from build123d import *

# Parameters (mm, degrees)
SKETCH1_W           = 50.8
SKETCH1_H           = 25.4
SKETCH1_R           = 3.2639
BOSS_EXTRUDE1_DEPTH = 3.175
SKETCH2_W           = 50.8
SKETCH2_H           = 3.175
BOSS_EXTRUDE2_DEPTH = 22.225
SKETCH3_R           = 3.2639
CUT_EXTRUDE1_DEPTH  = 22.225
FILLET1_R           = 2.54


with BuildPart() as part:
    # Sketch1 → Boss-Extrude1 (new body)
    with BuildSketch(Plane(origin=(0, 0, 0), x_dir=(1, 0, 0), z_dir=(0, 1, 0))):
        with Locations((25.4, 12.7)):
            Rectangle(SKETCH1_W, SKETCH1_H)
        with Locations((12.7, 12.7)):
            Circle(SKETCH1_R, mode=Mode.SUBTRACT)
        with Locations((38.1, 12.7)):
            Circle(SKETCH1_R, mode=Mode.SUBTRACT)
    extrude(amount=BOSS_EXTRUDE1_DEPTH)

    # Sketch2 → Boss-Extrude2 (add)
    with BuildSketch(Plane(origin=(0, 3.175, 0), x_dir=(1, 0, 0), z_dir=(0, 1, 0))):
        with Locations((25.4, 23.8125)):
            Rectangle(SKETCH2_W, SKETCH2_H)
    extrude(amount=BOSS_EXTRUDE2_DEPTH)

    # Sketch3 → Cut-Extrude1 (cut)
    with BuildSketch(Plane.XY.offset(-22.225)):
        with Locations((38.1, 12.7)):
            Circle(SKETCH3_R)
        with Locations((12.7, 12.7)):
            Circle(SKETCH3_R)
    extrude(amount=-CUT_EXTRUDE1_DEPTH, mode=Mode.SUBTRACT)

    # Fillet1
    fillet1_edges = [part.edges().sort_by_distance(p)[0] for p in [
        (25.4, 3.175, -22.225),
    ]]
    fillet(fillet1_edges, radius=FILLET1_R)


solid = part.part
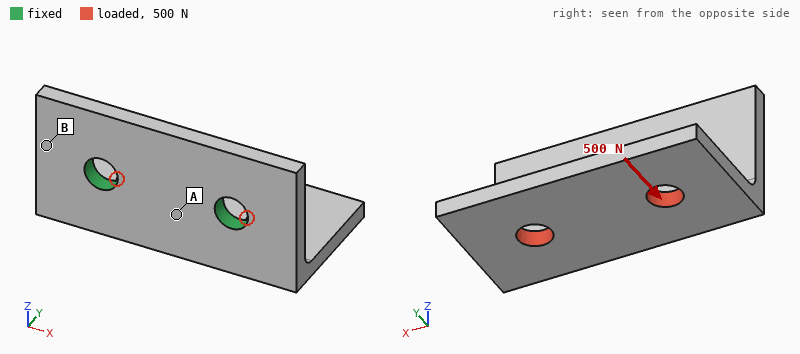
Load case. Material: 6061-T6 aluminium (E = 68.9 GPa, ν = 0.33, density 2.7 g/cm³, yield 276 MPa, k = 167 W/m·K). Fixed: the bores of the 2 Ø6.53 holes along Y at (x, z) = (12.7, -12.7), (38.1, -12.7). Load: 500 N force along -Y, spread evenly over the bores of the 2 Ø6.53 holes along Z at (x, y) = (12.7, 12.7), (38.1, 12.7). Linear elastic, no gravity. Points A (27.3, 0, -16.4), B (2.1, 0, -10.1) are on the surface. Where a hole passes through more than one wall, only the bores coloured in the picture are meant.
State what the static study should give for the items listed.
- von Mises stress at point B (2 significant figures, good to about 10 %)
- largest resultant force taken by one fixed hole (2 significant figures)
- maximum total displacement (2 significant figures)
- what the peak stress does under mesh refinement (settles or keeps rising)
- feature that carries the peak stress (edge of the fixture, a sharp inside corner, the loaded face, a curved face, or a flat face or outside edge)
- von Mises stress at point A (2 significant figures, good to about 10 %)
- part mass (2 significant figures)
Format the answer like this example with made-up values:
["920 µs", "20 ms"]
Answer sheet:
["9.0 MPa", "250 N", "61 µm", "keeps rising", "edge of the fixture", "20 MPa", "20 g"]
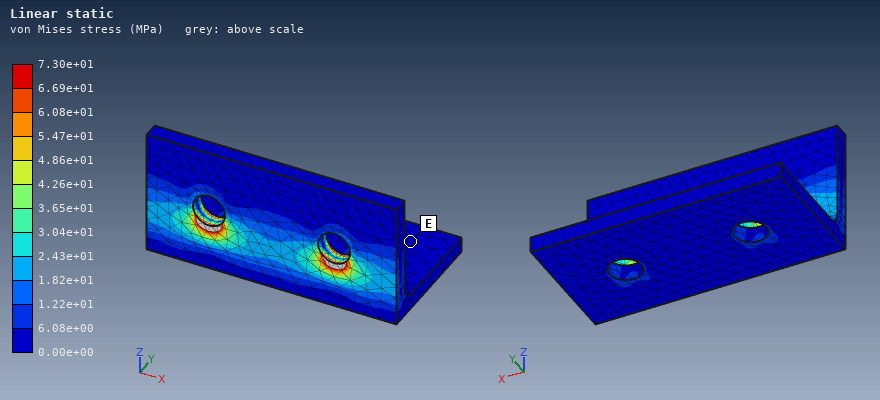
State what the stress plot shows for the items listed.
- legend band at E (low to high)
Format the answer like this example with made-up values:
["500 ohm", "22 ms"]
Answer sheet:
["0.00e+00 to 6.08e+00 MPa"]
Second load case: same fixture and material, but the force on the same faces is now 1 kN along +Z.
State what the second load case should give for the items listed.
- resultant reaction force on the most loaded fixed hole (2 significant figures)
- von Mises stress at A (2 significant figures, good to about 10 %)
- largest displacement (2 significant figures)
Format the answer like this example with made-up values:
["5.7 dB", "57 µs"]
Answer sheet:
["500 N", "78 MPa", "0.32 mm"]
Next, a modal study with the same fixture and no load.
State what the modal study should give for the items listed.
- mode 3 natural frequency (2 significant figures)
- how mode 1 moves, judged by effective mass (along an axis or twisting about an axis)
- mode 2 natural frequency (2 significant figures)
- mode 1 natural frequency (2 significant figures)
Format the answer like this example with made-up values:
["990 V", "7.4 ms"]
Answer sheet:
["8700 Hz", "along Z", "5000 Hz", "3100 Hz"]
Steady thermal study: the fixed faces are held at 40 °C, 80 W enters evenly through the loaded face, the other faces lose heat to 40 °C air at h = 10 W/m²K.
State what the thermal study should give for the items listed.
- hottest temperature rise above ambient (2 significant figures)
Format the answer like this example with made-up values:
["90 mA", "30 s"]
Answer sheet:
["72 K"]
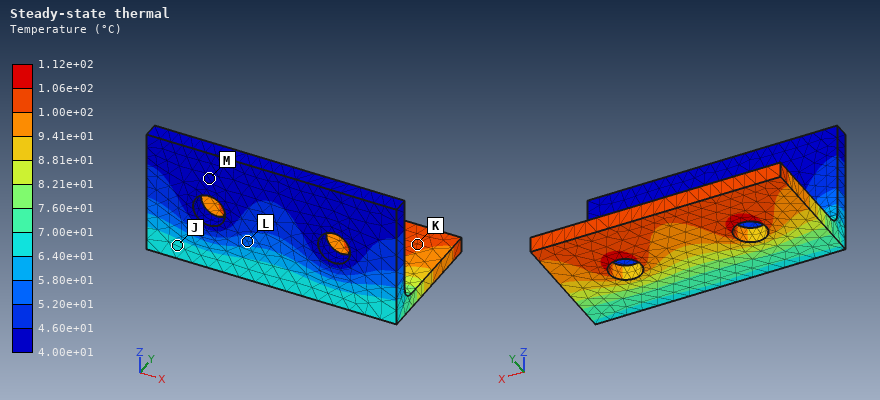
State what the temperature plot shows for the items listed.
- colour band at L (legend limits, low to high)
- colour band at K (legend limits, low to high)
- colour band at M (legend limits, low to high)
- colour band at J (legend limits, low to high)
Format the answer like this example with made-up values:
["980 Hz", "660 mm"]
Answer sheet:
["5.20e+01 to 5.80e+01 °C", "1.00e+02 to 1.06e+02 °C", "4.00e+01 to 4.60e+01 °C", "6.40e+01 to 7.00e+01 °C"]
